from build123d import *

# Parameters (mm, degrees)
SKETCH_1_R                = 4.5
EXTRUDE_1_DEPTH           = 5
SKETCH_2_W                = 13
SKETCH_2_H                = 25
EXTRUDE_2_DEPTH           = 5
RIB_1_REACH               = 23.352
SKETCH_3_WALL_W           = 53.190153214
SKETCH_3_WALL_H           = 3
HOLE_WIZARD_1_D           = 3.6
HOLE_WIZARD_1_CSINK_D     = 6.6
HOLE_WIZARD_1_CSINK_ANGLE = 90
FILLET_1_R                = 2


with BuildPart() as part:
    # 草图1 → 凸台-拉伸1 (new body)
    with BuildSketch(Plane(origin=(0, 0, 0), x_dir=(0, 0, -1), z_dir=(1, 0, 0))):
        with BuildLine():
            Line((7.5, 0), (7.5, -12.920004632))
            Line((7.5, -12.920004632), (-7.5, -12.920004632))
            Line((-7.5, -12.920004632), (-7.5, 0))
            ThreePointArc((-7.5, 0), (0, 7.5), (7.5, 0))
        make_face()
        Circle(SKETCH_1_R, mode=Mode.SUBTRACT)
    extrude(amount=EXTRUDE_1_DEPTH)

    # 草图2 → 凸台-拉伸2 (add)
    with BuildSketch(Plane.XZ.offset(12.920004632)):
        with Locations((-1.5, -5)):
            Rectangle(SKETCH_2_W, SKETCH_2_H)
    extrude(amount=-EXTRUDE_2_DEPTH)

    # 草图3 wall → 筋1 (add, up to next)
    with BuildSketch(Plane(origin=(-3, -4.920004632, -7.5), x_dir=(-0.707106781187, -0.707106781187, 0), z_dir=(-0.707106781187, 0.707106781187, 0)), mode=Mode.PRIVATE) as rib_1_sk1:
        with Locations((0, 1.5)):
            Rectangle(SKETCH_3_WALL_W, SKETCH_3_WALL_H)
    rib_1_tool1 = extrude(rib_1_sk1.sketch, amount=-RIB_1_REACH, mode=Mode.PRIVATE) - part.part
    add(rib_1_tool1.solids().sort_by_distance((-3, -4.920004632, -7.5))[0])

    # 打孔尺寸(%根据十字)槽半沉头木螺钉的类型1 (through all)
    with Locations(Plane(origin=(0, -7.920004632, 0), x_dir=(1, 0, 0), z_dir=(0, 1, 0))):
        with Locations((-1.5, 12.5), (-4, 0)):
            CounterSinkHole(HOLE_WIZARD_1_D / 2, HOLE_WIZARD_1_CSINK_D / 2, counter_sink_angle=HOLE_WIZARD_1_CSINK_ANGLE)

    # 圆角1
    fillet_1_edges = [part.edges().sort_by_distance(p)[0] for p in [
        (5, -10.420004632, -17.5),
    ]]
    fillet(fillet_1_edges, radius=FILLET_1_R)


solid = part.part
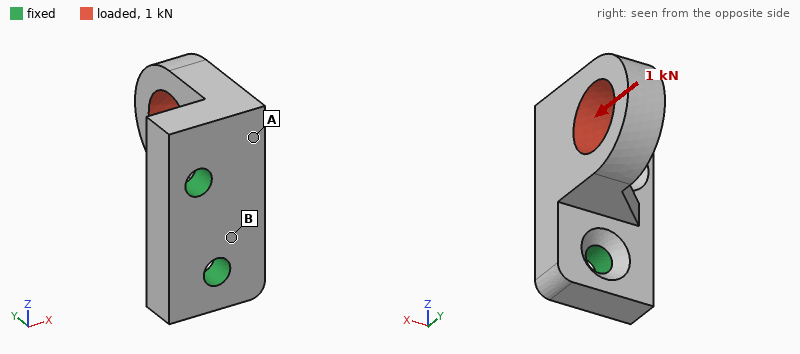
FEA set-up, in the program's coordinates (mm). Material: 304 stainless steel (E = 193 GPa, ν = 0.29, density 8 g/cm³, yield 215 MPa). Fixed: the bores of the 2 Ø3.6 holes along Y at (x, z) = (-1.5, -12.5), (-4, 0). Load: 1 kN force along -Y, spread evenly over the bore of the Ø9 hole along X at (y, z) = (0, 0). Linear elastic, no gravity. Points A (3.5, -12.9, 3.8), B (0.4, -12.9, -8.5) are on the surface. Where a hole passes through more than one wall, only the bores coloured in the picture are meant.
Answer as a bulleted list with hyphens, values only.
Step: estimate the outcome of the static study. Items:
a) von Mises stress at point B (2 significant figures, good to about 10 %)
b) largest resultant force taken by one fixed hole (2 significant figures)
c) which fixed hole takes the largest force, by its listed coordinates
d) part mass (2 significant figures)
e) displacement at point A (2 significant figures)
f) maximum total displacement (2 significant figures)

- 31 MPa
- 830 N
- (-4, 0)
- 18 g
- 6.6 µm
- 16 µm
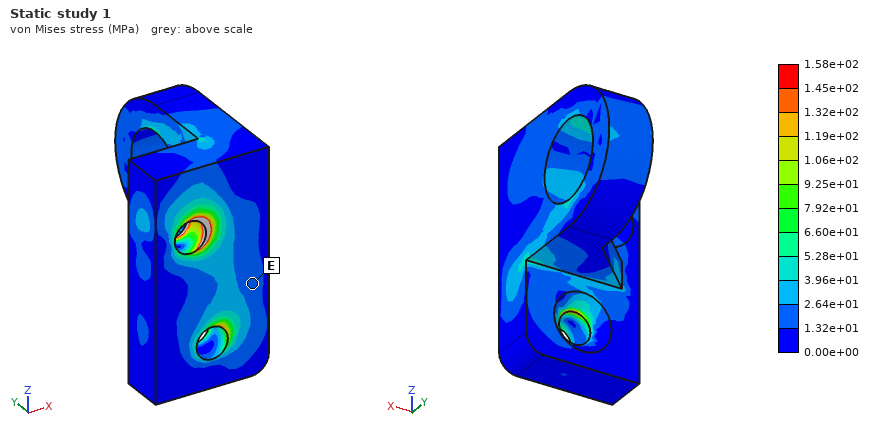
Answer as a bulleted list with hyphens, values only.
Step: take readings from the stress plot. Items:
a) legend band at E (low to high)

- 1.32e+01 to 2.64e+01 MPa
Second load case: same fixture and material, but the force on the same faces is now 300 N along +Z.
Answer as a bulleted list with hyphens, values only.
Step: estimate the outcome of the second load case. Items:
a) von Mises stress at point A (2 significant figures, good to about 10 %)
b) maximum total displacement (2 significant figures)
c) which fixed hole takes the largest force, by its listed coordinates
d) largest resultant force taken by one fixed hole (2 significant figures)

- 6.7 MPa
- 7.2 µm
- (-1.5, -12.5)
- 310 N
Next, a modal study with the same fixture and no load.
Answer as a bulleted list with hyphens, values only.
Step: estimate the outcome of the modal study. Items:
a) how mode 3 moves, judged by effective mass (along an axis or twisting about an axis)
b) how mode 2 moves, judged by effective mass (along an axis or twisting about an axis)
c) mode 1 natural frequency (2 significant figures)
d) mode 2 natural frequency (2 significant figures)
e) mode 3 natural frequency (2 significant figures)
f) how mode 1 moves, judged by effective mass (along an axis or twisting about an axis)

- along Y
- along Z
- 12 kHz
- 17 kHz
- 29 kHz
- along X
